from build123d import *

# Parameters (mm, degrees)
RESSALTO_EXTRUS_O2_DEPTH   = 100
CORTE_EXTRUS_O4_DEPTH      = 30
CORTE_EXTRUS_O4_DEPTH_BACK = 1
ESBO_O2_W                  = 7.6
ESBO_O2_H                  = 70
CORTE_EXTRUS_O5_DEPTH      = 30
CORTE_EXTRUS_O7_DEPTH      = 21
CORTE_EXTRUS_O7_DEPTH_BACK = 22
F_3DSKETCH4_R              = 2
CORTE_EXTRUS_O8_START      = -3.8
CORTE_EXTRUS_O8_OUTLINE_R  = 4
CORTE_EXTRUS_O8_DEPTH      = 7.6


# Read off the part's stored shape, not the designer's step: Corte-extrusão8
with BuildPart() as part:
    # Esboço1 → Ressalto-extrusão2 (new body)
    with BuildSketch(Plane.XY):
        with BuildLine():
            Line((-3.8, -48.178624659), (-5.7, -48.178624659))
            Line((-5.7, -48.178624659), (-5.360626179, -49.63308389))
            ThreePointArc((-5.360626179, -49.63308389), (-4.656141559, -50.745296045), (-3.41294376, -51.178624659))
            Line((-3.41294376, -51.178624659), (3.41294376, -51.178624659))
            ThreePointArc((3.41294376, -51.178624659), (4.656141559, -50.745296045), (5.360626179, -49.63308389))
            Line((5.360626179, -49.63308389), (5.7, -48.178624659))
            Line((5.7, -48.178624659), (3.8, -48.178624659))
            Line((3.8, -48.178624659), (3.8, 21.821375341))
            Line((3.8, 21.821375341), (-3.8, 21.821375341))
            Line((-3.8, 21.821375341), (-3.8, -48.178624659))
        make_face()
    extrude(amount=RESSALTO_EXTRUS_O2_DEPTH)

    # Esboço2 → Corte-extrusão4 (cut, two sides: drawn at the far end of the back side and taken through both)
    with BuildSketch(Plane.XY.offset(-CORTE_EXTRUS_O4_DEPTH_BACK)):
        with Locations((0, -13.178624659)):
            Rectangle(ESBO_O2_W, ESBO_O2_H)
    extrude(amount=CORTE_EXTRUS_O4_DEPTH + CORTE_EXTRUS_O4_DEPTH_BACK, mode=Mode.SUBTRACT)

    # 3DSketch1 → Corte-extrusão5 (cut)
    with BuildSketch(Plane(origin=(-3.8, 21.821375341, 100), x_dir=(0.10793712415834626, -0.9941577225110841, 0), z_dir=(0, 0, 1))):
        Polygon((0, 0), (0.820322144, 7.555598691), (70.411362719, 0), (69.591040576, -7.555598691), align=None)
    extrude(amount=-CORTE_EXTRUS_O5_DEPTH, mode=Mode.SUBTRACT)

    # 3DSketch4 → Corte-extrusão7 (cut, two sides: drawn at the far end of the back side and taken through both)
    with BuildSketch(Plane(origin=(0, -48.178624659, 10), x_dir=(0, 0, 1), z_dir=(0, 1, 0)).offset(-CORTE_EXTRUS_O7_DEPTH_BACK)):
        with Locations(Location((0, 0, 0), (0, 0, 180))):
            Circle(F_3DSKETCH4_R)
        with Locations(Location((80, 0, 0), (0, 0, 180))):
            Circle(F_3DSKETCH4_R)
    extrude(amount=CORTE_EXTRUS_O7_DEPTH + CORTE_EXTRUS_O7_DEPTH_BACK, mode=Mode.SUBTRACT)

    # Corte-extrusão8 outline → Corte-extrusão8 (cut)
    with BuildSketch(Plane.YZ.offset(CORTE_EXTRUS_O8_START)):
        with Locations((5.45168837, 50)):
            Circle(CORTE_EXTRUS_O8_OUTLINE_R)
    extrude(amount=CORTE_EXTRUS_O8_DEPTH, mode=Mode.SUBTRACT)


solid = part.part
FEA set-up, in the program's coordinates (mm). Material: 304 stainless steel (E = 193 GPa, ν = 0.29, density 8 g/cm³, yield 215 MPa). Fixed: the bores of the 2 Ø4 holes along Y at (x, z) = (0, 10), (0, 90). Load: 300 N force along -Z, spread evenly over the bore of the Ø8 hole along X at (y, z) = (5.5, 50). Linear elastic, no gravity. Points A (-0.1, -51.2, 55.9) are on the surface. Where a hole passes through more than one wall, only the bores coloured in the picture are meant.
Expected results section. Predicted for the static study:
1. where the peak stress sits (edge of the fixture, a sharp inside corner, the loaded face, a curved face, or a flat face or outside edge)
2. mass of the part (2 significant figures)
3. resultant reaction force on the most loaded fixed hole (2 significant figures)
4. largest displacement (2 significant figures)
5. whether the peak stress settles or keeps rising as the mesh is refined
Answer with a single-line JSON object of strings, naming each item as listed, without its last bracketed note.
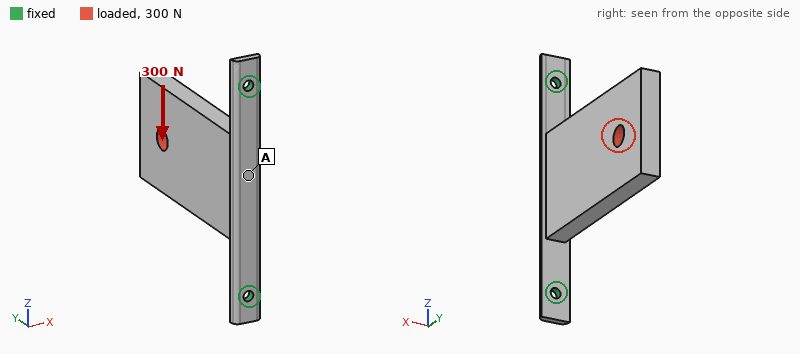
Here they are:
{"where the peak stress sits": "edge of the fixture", "mass of the part": "190 g", "resultant reaction force on the most loaded fixed hole": "320 N", "largest displacement": "0.13 mm", "whether the peak stress settles or keeps rising as the mesh is refined": "keeps rising"}
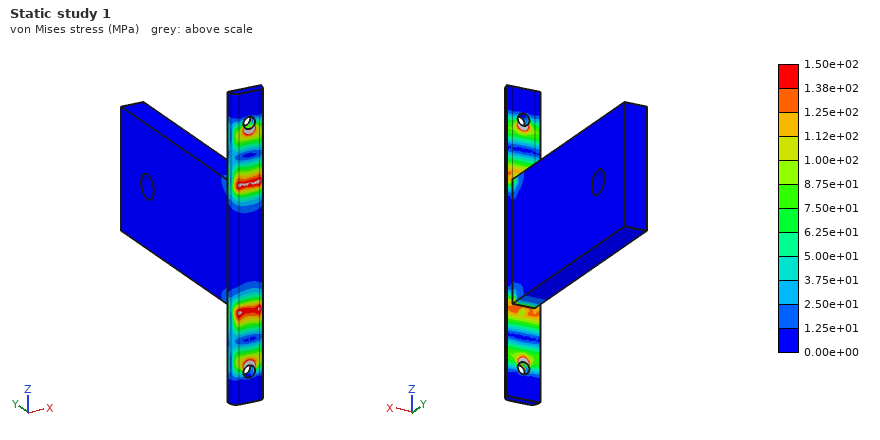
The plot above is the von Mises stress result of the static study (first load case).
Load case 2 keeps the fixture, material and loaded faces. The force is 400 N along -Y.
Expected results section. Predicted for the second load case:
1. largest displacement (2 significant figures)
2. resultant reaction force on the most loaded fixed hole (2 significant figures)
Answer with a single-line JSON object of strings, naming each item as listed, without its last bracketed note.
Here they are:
{"largest displacement": "36 µm", "resultant reaction force on the most loaded fixed hole": "240 N"}
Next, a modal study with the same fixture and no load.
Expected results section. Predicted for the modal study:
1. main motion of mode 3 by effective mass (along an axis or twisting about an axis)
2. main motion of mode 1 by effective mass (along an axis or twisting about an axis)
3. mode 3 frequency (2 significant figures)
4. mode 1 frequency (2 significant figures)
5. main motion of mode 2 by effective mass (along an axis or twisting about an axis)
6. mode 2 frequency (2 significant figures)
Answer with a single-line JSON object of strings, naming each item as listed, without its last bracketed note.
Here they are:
{"main motion of mode 3 by effective mass": "along Y", "main motion of mode 1 by effective mass": "along X", "mode 3 frequency": "1300 Hz", "mode 1 frequency": "230 Hz", "main motion of mode 2 by effective mass": "along Z", "mode 2 frequency": "870 Hz"}
